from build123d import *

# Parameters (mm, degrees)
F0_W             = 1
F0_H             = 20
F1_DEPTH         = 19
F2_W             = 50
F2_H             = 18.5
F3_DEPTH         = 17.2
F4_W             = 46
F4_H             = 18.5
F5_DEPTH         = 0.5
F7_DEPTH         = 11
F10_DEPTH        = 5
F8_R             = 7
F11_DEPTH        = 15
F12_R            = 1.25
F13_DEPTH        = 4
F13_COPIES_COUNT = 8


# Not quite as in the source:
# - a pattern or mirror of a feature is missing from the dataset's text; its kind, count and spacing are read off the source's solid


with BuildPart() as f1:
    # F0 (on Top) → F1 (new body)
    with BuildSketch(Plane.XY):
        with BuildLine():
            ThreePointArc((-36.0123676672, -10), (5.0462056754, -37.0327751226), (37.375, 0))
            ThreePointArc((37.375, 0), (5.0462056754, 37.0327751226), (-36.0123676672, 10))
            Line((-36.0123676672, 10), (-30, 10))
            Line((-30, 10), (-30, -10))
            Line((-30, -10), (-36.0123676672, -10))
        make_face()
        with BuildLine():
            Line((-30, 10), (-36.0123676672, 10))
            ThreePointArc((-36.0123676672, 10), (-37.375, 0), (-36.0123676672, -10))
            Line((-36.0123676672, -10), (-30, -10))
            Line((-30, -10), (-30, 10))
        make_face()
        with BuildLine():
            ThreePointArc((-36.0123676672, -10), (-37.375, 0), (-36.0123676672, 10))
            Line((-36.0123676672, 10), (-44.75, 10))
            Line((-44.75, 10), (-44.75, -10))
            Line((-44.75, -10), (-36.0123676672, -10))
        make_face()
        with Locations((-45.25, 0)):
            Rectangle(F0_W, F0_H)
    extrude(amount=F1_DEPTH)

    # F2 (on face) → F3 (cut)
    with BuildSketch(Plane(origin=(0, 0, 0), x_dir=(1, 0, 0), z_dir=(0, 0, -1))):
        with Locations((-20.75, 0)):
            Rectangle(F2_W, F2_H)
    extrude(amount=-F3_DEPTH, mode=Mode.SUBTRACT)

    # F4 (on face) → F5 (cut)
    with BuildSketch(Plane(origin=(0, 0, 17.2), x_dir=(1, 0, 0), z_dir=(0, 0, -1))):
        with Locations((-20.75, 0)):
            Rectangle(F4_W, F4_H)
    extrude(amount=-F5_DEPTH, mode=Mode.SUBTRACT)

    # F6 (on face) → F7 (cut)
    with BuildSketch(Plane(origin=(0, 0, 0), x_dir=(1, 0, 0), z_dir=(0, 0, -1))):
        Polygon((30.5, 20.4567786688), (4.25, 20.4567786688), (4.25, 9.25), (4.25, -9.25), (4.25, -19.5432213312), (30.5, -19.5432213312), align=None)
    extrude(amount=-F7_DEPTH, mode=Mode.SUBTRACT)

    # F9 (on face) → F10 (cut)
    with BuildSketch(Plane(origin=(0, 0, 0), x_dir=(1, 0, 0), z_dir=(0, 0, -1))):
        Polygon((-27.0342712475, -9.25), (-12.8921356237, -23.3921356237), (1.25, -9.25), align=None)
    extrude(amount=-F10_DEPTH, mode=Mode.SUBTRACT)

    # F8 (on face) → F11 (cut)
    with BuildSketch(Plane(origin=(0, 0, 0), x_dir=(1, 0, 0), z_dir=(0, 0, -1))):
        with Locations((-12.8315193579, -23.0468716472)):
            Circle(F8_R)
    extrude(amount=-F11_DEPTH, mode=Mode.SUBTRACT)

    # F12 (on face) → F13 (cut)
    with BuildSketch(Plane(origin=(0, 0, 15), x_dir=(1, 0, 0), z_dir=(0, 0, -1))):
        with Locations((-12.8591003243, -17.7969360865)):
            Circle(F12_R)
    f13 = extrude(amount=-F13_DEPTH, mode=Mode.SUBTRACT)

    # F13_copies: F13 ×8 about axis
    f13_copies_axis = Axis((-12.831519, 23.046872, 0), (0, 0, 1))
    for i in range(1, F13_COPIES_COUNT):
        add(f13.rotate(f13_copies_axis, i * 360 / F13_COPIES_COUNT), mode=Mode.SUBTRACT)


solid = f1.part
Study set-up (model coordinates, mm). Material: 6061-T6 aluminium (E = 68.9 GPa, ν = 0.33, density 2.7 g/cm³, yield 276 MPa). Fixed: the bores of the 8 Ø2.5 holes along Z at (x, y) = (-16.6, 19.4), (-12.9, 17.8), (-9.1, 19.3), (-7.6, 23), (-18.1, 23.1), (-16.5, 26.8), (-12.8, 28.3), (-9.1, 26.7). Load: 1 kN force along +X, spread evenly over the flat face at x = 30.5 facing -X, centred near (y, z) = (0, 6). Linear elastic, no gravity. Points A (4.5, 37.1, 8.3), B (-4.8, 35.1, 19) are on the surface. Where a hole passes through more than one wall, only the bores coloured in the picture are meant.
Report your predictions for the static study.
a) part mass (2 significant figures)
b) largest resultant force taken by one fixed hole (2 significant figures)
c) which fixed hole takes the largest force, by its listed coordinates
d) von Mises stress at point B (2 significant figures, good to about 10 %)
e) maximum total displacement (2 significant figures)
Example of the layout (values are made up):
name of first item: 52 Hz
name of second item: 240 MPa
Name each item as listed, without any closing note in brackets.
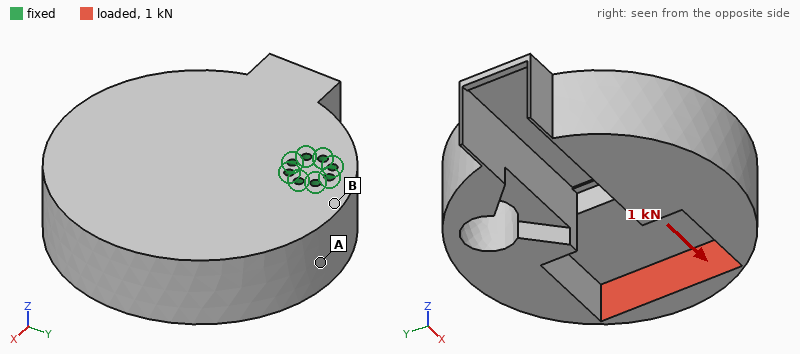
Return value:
part mass: 150 g
largest resultant force taken by one fixed hole: 770 N
which fixed hole takes the largest force, by its listed coordinates: (-12.9, 17.8)
von Mises stress at point B: 15 MPa
maximum total displacement: 0.10 mm
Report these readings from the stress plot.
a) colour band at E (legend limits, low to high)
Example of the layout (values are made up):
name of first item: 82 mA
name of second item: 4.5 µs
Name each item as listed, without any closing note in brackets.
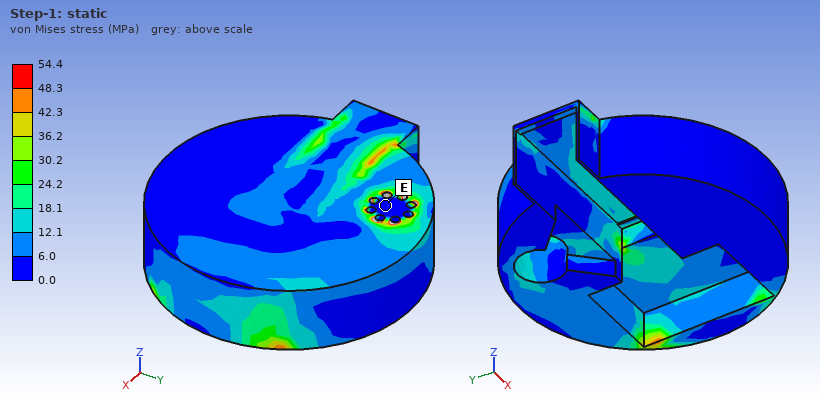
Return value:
colour band at E: 0.0 to 6.0 MPa
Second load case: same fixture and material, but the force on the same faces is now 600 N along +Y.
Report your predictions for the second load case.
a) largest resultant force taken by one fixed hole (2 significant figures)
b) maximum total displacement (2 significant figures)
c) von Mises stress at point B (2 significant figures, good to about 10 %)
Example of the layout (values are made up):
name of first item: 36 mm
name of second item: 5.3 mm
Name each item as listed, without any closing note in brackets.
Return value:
largest resultant force taken by one fixed hole: 670 N
maximum total displacement: 57 µm
von Mises stress at point B: 9.6 MPa
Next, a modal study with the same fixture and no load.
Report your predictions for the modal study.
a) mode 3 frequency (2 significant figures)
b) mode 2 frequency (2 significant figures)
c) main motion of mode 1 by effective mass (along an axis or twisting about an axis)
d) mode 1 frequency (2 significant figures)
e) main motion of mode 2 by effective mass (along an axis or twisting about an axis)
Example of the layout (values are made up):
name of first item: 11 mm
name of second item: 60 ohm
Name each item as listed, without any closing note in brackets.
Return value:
mode 3 frequency: 2500 Hz
mode 2 frequency: 1600 Hz
main motion of mode 1 by effective mass: along Z
mode 1 frequency: 990 Hz
main motion of mode 2 by effective mass: along X
